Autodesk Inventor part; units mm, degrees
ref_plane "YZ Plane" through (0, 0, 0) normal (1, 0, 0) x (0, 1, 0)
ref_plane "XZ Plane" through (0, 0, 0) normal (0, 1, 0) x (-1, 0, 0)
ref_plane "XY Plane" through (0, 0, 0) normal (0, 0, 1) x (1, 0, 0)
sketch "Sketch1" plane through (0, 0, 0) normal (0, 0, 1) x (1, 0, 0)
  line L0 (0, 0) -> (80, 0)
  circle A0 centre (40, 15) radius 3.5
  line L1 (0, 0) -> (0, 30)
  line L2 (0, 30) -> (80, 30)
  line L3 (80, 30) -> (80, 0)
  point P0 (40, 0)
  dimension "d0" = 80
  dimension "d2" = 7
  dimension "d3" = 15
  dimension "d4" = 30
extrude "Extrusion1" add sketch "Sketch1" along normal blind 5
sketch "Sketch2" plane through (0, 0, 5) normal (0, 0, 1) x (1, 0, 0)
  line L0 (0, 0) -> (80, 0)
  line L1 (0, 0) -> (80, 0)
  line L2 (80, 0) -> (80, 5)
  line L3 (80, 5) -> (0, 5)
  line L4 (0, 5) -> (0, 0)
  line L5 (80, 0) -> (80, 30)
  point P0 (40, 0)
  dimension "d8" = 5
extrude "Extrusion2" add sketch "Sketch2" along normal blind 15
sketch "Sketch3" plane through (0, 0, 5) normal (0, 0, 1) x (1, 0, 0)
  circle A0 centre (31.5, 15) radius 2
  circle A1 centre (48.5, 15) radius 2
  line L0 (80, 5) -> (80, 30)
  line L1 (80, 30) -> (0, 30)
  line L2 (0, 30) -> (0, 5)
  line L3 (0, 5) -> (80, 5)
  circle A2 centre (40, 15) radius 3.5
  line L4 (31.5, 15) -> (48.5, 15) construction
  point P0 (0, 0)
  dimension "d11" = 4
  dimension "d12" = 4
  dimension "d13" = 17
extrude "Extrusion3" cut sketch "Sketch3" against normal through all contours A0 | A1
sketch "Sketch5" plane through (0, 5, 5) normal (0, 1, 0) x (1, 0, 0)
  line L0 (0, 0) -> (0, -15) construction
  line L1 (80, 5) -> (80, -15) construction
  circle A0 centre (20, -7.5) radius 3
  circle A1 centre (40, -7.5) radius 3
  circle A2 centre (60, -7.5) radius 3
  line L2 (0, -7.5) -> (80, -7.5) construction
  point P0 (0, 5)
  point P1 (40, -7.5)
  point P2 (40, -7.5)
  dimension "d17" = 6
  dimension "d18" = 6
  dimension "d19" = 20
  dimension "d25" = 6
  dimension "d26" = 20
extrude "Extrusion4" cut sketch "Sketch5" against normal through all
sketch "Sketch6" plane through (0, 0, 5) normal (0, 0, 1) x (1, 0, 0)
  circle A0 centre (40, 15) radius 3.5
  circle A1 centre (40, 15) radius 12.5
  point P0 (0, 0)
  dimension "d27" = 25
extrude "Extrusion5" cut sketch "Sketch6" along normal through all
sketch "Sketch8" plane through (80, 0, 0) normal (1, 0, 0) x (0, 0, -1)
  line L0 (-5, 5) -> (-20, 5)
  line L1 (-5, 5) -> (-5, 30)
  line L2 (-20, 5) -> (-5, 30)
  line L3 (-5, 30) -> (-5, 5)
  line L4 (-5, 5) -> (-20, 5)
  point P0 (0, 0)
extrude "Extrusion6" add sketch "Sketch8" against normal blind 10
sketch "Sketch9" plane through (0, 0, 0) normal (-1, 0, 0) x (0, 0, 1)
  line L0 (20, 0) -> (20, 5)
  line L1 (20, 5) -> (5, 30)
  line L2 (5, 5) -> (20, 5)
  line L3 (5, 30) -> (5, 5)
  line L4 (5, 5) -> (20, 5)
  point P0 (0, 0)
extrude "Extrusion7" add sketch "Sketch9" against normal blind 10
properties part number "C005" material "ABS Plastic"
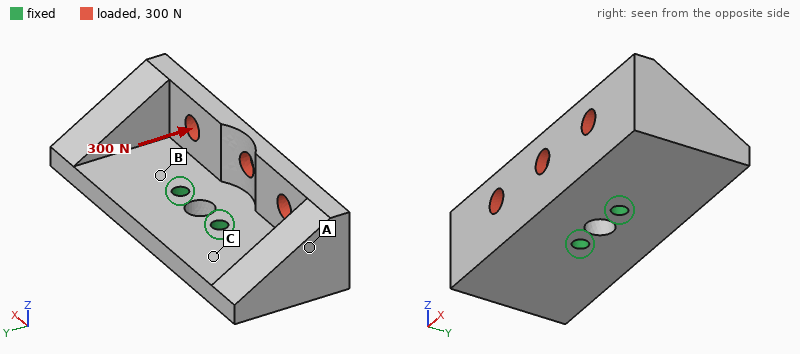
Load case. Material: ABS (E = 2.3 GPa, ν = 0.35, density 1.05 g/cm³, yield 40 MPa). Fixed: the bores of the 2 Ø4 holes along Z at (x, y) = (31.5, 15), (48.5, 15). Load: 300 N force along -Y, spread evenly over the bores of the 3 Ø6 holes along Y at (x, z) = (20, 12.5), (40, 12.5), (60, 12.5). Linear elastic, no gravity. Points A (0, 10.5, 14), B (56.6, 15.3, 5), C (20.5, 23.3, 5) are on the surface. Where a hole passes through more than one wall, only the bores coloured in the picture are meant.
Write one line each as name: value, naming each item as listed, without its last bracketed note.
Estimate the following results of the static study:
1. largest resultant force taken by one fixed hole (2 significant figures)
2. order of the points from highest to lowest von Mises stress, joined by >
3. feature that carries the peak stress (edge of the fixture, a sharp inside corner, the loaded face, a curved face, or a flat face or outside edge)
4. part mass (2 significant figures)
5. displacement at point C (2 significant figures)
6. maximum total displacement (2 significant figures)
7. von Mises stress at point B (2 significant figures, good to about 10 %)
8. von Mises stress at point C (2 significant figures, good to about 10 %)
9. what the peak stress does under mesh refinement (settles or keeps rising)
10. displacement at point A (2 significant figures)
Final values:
largest resultant force taken by one fixed hole: 150 N
order of the points from highest to lowest von Mises stress, joined by >: B > C > A
feature that carries the peak stress: edge of the fixture
part mass: 22 g
displacement at point C: 0.13 mm
maximum total displacement: 0.58 mm
von Mises stress at point B: 6.9 MPa
von Mises stress at point C: 4.8 MPa
what the peak stress does under mesh refinement: keeps rising
displacement at point A: 0.26 mm
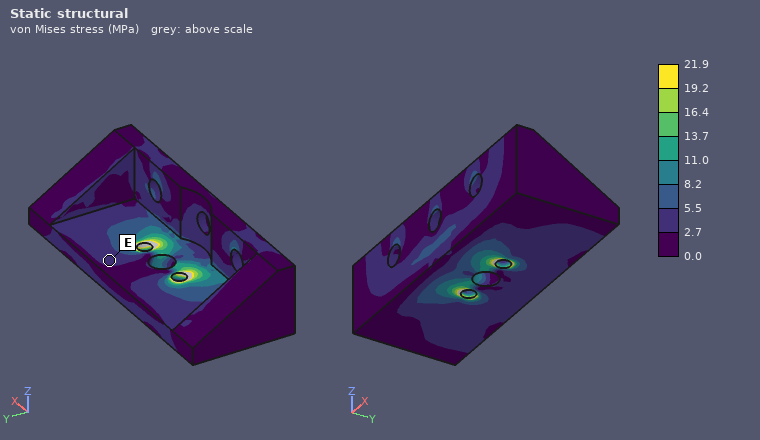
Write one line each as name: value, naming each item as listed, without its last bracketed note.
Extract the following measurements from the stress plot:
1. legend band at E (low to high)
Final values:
legend band at E: 2.7 to 5.5 MPa
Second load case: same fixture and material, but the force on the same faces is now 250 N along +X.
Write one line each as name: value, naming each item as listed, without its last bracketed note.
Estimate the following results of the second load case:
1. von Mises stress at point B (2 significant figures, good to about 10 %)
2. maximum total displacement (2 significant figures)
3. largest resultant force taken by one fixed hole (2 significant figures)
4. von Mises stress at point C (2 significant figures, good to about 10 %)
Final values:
von Mises stress at point B: 4.3 MPa
maximum total displacement: 0.40 mm
largest resultant force taken by one fixed hole: 210 N
von Mises stress at point C: 2.7 MPa
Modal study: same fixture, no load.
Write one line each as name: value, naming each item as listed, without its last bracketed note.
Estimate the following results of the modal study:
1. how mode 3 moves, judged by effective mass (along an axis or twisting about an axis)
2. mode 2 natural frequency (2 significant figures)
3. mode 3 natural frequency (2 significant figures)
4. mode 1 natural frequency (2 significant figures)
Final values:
how mode 3 moves, judged by effective mass: along Z
mode 2 natural frequency: 1200 Hz
mode 3 natural frequency: 1500 Hz
mode 1 natural frequency: 860 Hz
